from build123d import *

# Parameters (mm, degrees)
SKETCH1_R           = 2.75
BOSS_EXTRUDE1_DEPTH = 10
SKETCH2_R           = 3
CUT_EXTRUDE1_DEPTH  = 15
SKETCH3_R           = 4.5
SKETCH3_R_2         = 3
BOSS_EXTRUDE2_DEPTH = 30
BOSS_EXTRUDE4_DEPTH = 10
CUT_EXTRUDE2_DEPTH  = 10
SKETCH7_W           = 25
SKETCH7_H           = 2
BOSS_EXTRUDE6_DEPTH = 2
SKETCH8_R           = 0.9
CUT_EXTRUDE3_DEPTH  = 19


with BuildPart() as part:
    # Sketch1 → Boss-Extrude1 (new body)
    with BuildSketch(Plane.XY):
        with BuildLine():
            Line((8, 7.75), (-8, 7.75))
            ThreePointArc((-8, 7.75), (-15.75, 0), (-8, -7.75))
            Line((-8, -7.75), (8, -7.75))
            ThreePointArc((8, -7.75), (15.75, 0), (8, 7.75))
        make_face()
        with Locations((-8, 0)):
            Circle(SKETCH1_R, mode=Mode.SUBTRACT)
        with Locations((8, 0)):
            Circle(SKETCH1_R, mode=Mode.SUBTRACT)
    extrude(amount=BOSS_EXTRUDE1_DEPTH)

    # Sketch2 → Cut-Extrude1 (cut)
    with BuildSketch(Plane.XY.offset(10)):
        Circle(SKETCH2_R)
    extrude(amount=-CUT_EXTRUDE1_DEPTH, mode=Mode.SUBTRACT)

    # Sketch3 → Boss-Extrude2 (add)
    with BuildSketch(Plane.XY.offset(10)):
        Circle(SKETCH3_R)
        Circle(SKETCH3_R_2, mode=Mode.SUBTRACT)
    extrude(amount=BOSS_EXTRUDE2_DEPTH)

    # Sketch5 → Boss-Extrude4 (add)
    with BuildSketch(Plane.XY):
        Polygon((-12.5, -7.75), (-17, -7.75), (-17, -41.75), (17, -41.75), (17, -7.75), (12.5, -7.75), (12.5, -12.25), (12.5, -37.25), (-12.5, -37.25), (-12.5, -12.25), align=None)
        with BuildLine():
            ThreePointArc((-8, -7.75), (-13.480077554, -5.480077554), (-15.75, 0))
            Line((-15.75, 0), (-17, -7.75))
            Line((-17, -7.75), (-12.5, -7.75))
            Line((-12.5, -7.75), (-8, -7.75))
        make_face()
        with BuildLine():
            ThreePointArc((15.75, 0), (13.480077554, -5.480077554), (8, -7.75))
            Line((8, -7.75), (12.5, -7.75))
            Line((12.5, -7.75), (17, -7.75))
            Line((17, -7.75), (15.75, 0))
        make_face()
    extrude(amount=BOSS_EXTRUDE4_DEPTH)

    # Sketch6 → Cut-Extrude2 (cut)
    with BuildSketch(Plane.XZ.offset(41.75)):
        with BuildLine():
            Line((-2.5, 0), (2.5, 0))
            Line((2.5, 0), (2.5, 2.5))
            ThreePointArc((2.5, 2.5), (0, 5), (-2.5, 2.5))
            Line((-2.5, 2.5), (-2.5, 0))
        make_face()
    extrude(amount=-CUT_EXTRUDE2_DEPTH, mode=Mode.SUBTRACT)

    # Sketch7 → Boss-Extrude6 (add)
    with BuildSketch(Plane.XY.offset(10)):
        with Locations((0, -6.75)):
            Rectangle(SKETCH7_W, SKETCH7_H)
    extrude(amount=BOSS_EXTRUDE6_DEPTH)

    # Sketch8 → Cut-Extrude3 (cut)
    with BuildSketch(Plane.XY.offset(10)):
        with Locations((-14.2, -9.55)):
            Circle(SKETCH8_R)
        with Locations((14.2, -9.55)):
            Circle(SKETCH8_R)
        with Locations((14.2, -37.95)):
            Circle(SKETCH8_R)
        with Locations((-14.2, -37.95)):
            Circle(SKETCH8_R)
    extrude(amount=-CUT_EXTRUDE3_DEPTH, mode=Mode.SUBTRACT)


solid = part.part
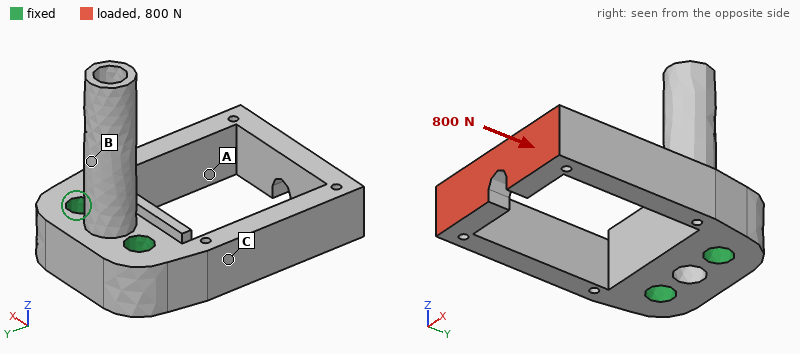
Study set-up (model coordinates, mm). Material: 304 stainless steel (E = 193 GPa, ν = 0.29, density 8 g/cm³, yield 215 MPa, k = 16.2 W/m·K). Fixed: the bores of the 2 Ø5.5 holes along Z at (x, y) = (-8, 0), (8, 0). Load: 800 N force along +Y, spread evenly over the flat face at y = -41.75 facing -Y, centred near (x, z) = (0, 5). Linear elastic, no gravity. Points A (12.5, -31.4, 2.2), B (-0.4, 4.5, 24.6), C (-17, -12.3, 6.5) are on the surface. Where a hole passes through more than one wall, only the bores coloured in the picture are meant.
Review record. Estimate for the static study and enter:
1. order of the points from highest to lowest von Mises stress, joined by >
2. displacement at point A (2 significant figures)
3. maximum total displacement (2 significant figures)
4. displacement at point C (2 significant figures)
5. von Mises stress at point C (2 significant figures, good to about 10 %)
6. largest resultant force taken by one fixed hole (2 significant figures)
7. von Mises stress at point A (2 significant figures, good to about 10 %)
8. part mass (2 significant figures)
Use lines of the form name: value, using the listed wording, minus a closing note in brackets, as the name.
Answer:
order of the points from highest to lowest von Mises stress, joined by >: A > C > B
displacement at point A: 4.5 µm
maximum total displacement: 12 µm
displacement at point C: 2.3 µm
von Mises stress at point C: 13 MPa
largest resultant force taken by one fixed hole: 400 N
von Mises stress at point A: 32 MPa
part mass: 73 g
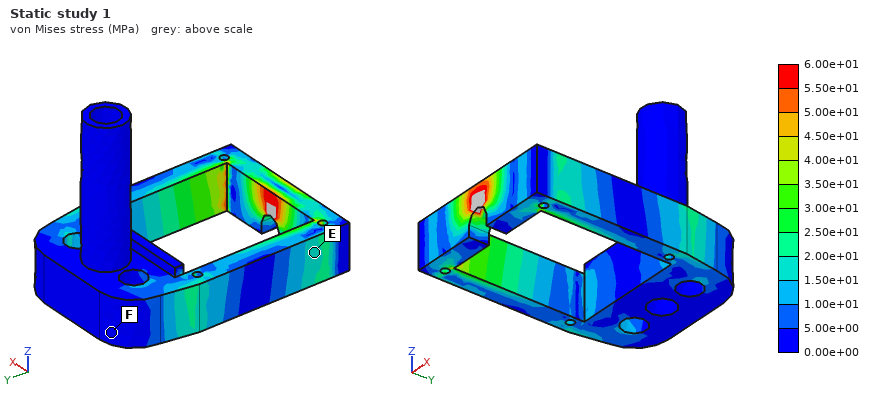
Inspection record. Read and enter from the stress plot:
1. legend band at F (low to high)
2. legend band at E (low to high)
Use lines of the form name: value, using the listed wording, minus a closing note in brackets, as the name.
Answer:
legend band at F: 0.00e+00 to 5.00e+00 MPa
legend band at E: 1.50e+01 to 2.00e+01 MPa
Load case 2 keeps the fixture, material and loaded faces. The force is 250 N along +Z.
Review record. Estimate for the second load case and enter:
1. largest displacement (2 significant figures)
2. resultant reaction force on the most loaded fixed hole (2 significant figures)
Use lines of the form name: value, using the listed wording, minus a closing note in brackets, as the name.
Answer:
largest displacement: 48 µm
resultant reaction force on the most loaded fixed hole: 130 N
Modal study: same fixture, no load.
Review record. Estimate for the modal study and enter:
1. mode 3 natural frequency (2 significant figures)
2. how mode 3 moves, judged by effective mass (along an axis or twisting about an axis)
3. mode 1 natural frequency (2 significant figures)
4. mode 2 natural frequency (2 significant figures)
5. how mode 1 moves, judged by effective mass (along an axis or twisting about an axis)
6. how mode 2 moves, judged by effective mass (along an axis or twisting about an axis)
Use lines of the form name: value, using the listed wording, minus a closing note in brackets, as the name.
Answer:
mode 3 natural frequency: 5500 Hz
how mode 3 moves, judged by effective mass: twisting about Y
mode 1 natural frequency: 2800 Hz
mode 2 natural frequency: 3200 Hz
how mode 1 moves, judged by effective mass: along X
how mode 2 moves, judged by effective mass: along Z
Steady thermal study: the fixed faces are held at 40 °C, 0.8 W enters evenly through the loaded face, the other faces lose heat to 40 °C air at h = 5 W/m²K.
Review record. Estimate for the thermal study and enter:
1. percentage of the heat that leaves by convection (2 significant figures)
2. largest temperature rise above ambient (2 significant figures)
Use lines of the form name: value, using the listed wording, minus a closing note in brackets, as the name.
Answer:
percentage of the heat that leaves by convection: 20 %
largest temperature rise above ambient: 21 K
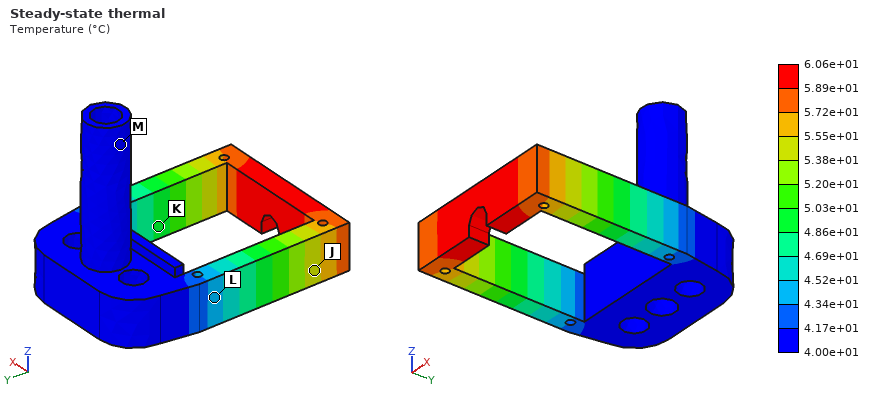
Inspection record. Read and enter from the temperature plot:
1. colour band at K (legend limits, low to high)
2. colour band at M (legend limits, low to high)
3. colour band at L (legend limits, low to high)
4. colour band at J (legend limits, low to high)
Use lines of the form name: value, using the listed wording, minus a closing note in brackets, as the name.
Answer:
colour band at K: 4.86e+01 to 5.03e+01 °C
colour band at M: 4.00e+01 to 4.17e+01 °C
colour band at L: 4.34e+01 to 4.52e+01 °C
colour band at J: 5.38e+01 to 5.55e+01 °C
